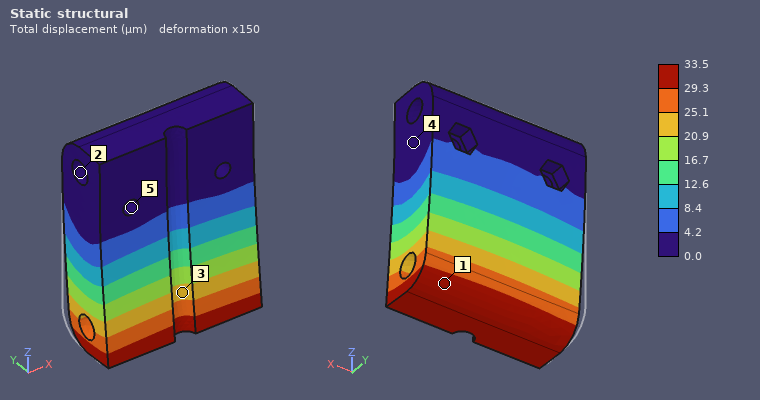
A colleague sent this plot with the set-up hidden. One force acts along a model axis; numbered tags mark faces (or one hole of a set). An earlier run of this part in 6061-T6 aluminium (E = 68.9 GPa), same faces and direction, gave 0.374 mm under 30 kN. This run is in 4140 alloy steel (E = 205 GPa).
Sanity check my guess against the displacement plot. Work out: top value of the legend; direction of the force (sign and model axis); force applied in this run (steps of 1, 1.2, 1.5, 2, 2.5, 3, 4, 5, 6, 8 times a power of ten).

33.5 µm
-Y
8 kN
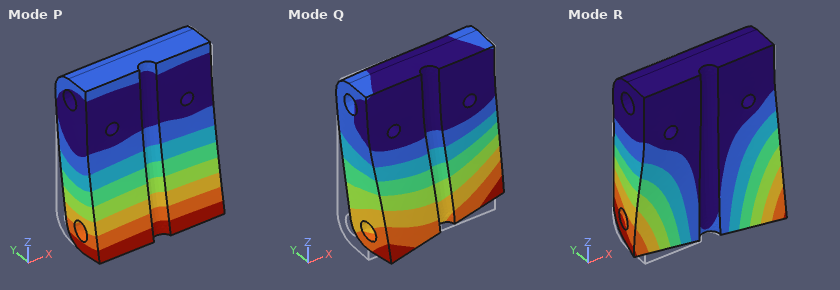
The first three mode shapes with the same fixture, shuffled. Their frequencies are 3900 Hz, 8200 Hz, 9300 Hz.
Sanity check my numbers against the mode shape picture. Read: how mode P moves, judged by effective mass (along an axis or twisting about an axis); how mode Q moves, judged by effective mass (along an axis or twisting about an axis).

along Y
along X
